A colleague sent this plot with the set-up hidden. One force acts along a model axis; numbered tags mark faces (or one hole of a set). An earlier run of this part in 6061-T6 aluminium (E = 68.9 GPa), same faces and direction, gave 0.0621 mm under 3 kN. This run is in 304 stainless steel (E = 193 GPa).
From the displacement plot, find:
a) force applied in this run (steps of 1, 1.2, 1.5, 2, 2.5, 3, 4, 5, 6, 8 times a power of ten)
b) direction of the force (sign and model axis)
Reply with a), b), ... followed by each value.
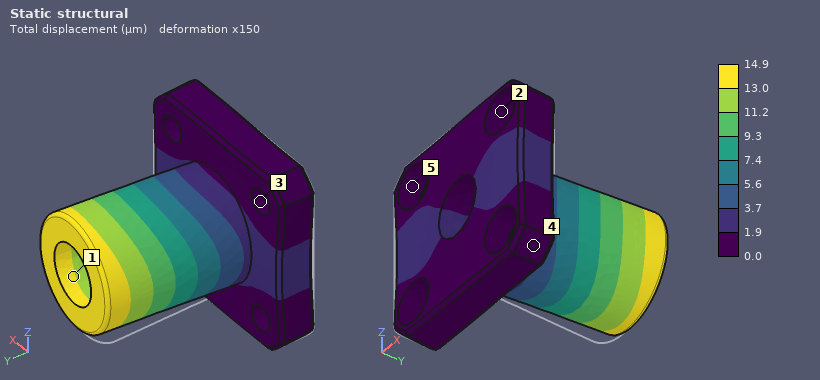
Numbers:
a) 2 kN
b) +X
